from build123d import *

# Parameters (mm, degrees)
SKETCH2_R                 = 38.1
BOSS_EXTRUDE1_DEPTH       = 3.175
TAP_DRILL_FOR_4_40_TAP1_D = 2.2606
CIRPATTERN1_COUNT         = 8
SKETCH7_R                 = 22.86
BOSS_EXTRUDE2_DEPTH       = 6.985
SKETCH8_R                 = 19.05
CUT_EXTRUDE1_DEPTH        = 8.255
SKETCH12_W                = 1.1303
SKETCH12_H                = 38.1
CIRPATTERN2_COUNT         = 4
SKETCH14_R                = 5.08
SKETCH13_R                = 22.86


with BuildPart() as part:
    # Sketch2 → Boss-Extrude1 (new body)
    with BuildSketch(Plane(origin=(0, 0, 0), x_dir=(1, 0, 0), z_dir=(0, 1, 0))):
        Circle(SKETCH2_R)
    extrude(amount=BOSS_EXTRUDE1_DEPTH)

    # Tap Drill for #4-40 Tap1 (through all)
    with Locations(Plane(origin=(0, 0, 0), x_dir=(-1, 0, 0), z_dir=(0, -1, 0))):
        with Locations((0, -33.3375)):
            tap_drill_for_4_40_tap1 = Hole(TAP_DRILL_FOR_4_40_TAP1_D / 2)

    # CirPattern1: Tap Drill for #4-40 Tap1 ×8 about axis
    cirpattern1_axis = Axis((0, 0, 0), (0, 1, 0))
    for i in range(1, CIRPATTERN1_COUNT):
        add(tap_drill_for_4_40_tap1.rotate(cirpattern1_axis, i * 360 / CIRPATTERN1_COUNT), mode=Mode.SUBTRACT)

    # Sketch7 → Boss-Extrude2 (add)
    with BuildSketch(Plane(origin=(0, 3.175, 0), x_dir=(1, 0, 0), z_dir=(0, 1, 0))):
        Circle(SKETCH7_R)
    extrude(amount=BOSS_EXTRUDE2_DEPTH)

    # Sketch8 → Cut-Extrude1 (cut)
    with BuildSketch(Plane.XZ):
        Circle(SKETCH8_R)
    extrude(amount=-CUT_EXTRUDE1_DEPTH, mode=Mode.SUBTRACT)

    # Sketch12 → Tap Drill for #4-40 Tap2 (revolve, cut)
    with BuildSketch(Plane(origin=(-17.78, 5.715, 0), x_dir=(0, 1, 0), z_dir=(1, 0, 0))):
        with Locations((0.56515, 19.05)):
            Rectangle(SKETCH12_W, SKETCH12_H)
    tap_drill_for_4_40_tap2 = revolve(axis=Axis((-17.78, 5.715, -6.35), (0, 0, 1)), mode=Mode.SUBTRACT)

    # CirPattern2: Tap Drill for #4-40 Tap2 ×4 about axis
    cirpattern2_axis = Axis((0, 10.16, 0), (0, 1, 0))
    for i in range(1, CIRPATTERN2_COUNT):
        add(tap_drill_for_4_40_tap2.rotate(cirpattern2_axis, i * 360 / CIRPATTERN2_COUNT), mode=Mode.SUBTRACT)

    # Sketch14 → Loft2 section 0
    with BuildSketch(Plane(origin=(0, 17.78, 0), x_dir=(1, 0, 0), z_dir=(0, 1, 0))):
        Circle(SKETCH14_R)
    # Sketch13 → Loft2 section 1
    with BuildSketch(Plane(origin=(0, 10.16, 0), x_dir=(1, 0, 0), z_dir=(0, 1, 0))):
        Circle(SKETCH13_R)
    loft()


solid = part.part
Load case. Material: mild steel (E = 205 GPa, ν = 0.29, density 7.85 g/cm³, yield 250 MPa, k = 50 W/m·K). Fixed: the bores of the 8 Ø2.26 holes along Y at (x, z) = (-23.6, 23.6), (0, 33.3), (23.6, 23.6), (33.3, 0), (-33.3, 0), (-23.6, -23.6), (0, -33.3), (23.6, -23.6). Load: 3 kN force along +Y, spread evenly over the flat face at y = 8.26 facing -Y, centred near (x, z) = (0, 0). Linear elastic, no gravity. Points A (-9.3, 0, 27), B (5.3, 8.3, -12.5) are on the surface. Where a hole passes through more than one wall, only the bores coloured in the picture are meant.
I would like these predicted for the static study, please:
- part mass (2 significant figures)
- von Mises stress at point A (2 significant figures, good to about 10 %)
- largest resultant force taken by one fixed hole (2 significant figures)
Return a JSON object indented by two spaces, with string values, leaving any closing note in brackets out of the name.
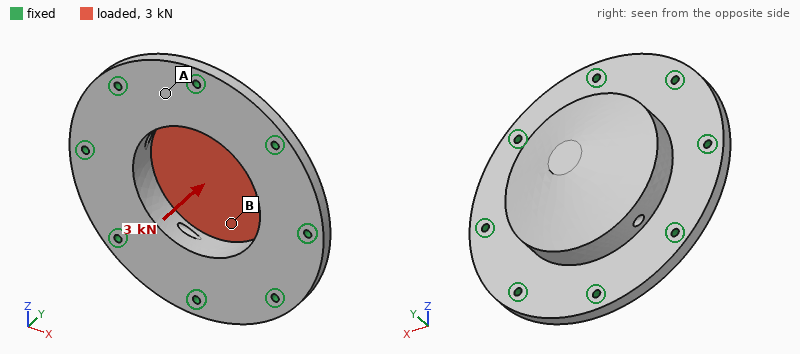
{
  "part mass": "170 g",
  "von Mises stress at point A": "21 MPa",
  "largest resultant force taken by one fixed hole": "510 N"
}
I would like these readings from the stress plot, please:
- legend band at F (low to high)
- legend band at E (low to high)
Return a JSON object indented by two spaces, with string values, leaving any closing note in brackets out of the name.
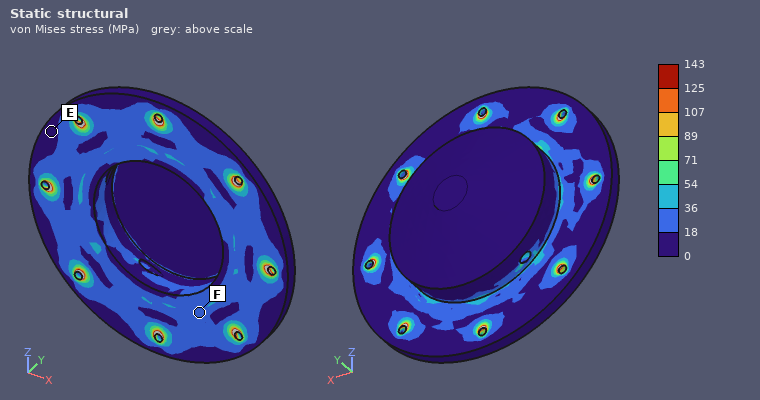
{
  "legend band at F": "18 to 36 MPa",
  "legend band at E": "0 to 18 MPa"
}
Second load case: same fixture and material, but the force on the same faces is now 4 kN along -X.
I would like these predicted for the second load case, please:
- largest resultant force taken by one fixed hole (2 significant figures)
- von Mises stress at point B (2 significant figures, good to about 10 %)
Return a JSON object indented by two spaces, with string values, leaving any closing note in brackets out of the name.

{
  "largest resultant force taken by one fixed hole": "650 N",
  "von Mises stress at point B": "17 MPa"
}
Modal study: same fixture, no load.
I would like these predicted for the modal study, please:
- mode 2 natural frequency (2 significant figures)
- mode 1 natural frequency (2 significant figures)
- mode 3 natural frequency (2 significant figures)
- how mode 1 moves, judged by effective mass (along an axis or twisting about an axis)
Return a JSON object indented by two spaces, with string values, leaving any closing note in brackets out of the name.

{
  "mode 2 natural frequency": "11 kHz",
  "mode 1 natural frequency": "8100 Hz",
  "mode 3 natural frequency": "11 kHz",
  "how mode 1 moves, judged by effective mass": "along Y"
}
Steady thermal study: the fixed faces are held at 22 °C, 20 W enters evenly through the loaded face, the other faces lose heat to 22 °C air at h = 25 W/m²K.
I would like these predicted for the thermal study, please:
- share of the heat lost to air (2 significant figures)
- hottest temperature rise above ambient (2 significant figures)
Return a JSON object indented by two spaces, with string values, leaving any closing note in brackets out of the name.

{
  "share of the heat lost to air": "12 %",
  "hottest temperature rise above ambient": "24 K"
}
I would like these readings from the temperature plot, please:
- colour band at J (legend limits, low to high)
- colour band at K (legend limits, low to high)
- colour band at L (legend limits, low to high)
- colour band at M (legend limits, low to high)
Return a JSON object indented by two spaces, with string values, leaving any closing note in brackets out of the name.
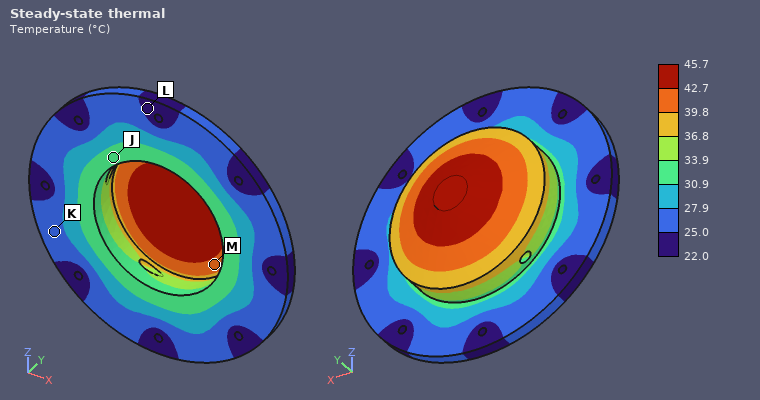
{
  "colour band at J": "30.9 to 33.9 °C",
  "colour band at K": "25.0 to 27.9 °C",
  "colour band at L": "22.0 to 25.0 °C",
  "colour band at M": "39.8 to 42.7 °C"
}
